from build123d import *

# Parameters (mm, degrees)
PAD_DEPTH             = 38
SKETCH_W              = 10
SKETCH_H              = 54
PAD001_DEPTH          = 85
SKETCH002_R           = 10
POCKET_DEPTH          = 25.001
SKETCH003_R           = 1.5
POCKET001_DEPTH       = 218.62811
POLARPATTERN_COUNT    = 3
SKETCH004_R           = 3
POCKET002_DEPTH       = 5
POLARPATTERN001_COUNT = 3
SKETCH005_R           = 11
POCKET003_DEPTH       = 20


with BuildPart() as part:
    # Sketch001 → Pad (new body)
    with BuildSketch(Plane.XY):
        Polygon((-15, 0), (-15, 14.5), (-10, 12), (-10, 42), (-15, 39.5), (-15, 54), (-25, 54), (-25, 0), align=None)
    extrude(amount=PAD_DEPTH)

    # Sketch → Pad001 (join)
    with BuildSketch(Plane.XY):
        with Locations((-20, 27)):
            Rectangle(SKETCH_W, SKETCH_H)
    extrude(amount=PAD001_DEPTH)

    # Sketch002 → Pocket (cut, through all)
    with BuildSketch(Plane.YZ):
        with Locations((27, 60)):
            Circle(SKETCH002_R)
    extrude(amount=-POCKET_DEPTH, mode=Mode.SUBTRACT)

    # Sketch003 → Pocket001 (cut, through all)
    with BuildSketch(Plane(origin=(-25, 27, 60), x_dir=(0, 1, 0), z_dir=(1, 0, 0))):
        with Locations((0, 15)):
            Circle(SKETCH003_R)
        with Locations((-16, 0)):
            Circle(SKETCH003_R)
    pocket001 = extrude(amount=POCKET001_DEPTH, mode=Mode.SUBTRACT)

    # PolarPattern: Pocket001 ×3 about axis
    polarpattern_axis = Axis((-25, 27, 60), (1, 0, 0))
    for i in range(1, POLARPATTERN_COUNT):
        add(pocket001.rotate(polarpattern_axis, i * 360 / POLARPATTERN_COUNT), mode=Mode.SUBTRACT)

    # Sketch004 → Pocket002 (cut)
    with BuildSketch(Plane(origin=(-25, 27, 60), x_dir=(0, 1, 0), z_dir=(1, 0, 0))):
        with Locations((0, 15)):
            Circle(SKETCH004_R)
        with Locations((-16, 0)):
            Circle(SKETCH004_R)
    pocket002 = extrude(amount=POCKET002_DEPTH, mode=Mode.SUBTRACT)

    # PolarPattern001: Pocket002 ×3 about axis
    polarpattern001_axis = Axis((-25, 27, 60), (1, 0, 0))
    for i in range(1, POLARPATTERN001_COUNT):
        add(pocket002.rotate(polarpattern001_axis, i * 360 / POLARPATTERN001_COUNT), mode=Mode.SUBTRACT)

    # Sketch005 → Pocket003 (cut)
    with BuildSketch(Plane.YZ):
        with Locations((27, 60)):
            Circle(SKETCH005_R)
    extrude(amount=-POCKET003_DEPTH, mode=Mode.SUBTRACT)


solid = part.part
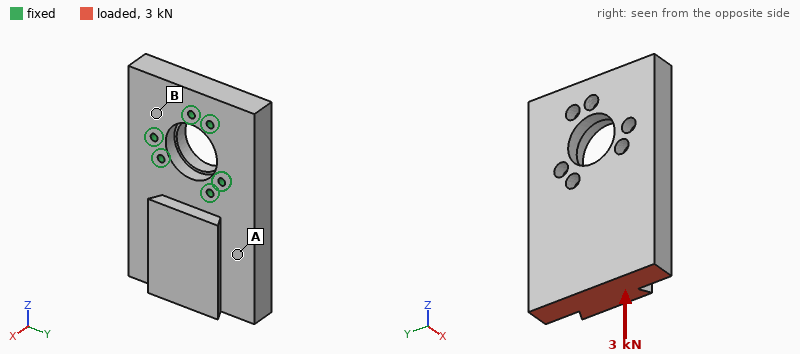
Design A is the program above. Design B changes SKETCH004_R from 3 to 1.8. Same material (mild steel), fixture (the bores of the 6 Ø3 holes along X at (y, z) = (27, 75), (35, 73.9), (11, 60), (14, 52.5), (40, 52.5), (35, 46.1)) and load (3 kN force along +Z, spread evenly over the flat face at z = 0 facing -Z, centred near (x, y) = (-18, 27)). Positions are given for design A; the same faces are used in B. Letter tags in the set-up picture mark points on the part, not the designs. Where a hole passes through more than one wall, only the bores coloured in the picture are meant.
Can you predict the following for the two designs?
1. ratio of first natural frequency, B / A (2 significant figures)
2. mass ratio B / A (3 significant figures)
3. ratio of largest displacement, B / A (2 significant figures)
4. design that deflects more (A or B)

1.1
1.01
1.2
B
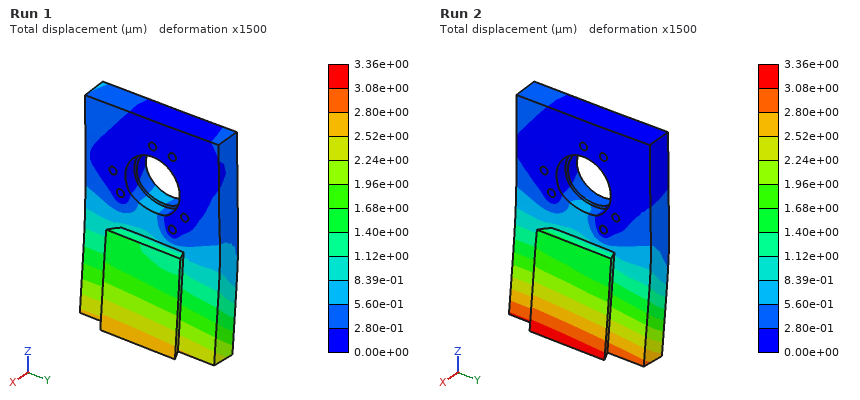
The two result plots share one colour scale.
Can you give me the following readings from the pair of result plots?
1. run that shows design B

Run 2
